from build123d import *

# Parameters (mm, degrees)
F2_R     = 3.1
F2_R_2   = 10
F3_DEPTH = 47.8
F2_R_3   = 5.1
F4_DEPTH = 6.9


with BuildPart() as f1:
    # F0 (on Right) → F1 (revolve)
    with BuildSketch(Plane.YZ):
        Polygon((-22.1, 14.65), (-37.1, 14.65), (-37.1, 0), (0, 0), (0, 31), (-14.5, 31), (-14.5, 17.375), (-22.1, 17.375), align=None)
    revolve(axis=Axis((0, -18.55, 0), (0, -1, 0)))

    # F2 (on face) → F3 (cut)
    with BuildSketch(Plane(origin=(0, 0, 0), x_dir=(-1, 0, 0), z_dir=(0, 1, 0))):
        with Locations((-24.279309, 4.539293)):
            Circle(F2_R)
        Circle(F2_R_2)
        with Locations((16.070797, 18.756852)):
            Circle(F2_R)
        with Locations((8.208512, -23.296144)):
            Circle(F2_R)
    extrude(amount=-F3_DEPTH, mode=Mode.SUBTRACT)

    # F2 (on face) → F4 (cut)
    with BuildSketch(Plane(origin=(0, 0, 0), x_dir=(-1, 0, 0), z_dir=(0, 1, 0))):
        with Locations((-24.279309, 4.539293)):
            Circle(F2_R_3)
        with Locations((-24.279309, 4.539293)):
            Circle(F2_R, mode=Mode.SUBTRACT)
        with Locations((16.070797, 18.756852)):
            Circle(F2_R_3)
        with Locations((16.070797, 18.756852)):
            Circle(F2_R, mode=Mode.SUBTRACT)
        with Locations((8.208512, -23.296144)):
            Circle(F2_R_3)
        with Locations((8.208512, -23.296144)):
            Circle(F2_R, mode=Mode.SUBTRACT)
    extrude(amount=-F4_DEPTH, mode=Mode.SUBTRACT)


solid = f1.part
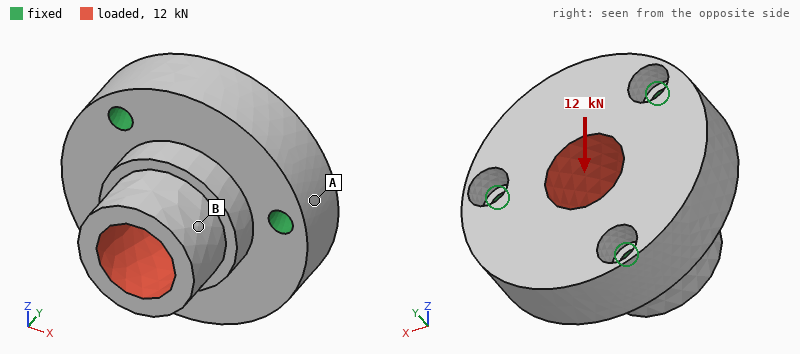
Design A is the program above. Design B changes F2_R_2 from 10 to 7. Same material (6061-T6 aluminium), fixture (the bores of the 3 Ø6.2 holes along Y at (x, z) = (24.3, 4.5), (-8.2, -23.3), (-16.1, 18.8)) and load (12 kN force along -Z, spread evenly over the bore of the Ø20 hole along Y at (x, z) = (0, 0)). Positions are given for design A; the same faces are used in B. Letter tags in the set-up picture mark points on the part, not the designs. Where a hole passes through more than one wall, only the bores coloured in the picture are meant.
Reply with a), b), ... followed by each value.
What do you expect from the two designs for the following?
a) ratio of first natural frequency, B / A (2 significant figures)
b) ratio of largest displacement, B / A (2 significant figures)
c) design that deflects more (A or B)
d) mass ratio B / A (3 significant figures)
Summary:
a) 1.0
b) 0.79
c) A
d) 1.13
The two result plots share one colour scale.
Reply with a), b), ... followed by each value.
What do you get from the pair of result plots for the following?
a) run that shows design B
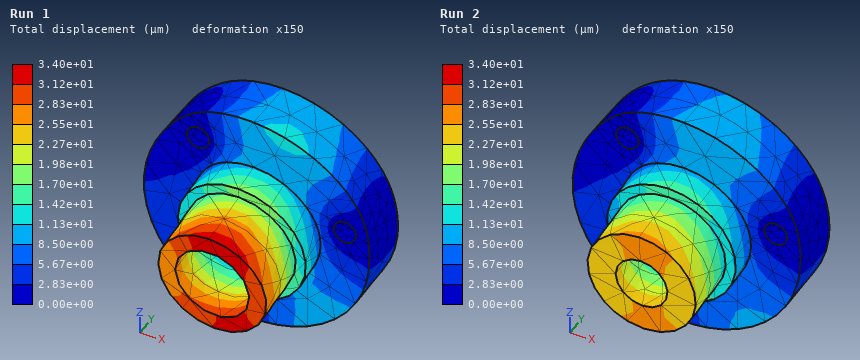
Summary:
a) Run 2
